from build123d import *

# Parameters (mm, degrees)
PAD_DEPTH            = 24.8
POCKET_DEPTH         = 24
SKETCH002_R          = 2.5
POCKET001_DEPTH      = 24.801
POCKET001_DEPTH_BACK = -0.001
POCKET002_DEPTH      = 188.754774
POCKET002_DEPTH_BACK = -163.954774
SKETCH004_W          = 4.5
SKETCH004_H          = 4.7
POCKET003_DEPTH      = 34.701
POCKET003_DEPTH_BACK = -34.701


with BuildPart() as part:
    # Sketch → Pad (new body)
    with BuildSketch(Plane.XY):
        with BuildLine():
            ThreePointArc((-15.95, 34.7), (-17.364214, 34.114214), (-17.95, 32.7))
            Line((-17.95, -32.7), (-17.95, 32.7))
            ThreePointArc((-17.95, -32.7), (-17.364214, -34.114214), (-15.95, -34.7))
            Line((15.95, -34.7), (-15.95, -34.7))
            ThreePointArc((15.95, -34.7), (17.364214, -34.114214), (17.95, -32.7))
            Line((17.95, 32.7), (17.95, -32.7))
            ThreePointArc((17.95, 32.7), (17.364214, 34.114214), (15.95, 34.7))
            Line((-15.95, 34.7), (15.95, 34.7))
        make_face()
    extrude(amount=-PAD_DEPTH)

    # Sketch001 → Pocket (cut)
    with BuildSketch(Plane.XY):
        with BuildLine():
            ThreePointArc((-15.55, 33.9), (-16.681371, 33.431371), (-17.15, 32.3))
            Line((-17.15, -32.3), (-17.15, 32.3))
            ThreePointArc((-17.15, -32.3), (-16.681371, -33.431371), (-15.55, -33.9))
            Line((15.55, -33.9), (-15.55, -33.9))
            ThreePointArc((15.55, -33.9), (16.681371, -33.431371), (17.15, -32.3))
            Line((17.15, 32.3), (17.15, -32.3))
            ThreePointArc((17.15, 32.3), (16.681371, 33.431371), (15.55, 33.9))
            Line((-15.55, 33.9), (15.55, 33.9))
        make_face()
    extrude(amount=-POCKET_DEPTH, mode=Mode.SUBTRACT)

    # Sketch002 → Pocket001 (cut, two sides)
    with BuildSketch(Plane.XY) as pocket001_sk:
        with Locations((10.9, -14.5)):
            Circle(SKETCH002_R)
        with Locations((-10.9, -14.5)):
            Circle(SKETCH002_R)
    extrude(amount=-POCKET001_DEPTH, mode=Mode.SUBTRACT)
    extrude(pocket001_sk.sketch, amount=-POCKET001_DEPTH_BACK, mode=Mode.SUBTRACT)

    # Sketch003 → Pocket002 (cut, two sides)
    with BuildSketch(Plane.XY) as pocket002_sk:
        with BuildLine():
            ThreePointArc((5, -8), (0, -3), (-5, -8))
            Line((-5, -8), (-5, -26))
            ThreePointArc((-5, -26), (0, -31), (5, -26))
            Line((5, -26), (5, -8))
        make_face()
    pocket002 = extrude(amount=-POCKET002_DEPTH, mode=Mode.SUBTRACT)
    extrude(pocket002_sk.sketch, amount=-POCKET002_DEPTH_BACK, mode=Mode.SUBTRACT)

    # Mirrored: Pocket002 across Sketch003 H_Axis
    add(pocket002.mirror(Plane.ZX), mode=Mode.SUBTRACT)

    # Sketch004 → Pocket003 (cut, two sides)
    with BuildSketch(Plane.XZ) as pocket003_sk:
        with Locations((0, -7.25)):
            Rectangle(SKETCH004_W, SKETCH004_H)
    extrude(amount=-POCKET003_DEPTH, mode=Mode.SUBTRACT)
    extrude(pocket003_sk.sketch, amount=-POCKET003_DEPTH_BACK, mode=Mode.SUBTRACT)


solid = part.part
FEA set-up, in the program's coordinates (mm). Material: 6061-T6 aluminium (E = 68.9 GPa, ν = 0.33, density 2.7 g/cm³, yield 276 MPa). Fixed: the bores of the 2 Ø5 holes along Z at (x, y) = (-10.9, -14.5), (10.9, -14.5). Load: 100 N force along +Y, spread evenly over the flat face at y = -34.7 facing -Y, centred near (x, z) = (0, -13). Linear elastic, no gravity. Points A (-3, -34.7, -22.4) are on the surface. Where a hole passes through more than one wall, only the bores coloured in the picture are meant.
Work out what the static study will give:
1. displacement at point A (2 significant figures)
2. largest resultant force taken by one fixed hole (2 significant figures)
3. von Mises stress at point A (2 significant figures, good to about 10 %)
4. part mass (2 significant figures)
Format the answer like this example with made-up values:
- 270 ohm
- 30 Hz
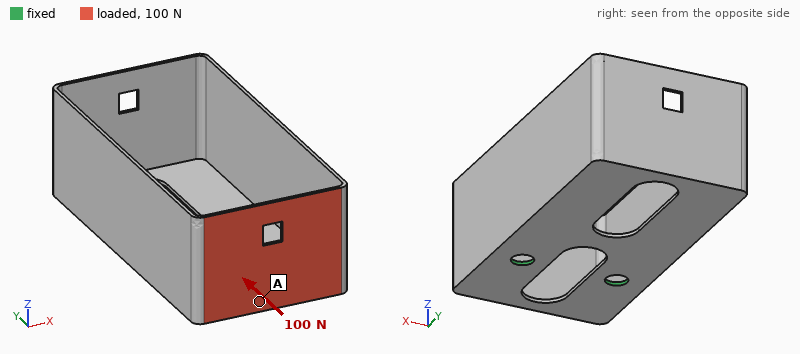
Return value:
- 0.31 mm
- 53 N
- 21 MPa
- 15 g
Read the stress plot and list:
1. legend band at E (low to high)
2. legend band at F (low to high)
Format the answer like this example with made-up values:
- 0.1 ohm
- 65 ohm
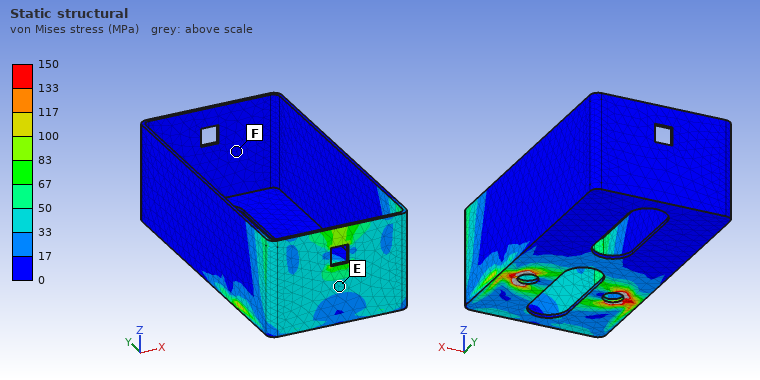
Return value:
- 33 to 50 MPa
- 0 to 17 MPa
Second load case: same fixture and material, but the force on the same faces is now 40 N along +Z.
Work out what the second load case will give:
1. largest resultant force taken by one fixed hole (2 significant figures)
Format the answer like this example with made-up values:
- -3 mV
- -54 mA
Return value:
- 21 N
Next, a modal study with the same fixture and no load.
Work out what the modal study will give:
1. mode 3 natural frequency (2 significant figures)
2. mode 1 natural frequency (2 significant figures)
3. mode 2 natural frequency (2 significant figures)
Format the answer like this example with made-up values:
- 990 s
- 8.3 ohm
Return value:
- 1300 Hz
- 380 Hz
- 580 Hz
